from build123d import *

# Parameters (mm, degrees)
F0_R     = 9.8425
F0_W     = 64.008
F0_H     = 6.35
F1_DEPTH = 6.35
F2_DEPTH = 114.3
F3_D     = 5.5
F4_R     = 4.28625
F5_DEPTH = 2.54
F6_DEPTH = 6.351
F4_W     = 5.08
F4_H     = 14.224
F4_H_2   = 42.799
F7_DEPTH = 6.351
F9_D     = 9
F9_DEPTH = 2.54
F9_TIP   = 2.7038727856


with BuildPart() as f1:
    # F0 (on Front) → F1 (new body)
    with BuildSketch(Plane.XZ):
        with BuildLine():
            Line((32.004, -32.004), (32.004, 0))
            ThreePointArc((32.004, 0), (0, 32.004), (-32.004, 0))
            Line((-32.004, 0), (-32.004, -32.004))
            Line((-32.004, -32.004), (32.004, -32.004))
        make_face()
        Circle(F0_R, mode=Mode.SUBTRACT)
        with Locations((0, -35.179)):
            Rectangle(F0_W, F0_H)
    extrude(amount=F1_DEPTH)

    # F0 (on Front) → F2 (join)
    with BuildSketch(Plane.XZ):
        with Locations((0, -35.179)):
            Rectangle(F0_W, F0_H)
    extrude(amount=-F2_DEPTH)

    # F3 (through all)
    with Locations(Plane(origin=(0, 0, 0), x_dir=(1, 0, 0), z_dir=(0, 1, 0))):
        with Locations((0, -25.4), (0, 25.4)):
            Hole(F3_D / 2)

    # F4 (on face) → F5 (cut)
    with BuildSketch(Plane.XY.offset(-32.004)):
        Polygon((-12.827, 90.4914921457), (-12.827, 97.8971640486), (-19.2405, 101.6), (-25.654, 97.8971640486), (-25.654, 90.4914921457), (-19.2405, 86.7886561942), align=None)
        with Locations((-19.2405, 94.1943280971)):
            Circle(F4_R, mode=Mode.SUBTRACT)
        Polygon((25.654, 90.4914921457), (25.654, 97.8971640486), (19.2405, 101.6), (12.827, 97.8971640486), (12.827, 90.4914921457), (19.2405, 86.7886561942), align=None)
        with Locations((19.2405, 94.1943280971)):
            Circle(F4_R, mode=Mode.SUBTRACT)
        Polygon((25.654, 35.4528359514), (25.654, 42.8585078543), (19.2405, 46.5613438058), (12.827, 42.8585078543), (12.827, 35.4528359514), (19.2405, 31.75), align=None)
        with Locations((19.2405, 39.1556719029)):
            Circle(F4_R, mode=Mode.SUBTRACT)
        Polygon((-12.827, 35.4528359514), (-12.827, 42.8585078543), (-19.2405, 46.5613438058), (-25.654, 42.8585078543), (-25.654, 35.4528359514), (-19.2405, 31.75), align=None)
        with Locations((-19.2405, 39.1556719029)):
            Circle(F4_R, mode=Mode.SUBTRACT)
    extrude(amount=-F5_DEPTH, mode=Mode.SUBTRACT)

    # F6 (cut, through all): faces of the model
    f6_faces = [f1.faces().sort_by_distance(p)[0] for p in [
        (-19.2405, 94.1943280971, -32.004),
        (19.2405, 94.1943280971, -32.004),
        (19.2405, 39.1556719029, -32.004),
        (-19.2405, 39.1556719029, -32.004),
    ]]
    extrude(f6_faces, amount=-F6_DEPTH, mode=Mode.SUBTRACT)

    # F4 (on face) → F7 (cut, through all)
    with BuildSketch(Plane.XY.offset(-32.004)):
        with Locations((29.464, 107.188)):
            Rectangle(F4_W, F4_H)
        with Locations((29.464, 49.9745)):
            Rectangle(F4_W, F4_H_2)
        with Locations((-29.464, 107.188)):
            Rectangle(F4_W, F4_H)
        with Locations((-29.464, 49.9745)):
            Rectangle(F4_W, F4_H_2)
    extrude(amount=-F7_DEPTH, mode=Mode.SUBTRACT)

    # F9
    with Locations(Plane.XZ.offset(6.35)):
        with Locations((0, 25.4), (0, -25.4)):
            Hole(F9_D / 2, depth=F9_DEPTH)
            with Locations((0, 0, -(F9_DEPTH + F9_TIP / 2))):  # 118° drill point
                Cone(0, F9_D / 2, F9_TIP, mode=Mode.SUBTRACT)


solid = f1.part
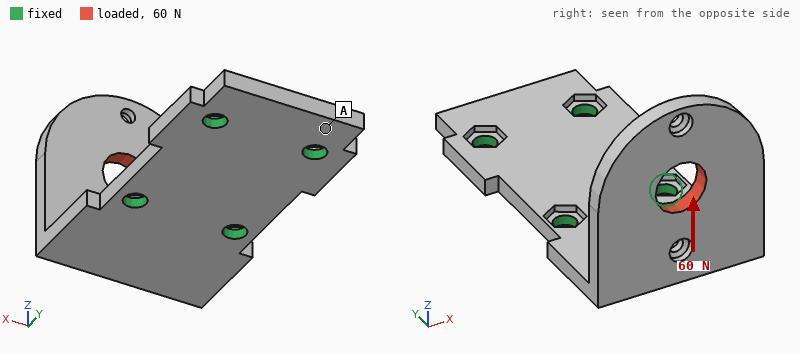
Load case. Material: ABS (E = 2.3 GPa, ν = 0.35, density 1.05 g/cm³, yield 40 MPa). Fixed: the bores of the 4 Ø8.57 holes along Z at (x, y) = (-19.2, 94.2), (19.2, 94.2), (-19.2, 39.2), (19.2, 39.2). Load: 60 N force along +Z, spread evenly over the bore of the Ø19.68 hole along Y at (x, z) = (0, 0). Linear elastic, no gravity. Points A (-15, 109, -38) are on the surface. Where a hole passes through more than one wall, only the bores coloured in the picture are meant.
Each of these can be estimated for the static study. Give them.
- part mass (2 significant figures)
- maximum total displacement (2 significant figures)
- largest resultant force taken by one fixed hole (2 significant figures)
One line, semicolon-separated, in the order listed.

67 g; 1.6 mm; 51 N
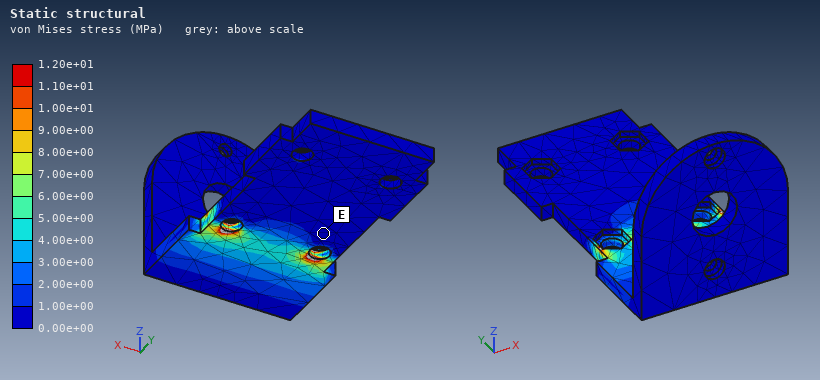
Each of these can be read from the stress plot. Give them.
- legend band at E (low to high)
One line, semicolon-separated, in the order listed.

0.00e+00 to 1.00e+00 MPa
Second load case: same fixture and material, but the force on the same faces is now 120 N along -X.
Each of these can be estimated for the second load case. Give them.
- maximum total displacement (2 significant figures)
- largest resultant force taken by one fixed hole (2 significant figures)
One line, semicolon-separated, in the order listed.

1.6 mm; 180 N
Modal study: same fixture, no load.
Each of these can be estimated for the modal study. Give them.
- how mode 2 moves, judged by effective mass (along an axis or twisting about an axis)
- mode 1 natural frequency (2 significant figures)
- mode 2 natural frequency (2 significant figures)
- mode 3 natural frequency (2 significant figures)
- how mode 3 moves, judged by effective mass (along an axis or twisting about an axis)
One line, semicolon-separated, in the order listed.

along X; 180 Hz; 340 Hz; 520 Hz; along Z
